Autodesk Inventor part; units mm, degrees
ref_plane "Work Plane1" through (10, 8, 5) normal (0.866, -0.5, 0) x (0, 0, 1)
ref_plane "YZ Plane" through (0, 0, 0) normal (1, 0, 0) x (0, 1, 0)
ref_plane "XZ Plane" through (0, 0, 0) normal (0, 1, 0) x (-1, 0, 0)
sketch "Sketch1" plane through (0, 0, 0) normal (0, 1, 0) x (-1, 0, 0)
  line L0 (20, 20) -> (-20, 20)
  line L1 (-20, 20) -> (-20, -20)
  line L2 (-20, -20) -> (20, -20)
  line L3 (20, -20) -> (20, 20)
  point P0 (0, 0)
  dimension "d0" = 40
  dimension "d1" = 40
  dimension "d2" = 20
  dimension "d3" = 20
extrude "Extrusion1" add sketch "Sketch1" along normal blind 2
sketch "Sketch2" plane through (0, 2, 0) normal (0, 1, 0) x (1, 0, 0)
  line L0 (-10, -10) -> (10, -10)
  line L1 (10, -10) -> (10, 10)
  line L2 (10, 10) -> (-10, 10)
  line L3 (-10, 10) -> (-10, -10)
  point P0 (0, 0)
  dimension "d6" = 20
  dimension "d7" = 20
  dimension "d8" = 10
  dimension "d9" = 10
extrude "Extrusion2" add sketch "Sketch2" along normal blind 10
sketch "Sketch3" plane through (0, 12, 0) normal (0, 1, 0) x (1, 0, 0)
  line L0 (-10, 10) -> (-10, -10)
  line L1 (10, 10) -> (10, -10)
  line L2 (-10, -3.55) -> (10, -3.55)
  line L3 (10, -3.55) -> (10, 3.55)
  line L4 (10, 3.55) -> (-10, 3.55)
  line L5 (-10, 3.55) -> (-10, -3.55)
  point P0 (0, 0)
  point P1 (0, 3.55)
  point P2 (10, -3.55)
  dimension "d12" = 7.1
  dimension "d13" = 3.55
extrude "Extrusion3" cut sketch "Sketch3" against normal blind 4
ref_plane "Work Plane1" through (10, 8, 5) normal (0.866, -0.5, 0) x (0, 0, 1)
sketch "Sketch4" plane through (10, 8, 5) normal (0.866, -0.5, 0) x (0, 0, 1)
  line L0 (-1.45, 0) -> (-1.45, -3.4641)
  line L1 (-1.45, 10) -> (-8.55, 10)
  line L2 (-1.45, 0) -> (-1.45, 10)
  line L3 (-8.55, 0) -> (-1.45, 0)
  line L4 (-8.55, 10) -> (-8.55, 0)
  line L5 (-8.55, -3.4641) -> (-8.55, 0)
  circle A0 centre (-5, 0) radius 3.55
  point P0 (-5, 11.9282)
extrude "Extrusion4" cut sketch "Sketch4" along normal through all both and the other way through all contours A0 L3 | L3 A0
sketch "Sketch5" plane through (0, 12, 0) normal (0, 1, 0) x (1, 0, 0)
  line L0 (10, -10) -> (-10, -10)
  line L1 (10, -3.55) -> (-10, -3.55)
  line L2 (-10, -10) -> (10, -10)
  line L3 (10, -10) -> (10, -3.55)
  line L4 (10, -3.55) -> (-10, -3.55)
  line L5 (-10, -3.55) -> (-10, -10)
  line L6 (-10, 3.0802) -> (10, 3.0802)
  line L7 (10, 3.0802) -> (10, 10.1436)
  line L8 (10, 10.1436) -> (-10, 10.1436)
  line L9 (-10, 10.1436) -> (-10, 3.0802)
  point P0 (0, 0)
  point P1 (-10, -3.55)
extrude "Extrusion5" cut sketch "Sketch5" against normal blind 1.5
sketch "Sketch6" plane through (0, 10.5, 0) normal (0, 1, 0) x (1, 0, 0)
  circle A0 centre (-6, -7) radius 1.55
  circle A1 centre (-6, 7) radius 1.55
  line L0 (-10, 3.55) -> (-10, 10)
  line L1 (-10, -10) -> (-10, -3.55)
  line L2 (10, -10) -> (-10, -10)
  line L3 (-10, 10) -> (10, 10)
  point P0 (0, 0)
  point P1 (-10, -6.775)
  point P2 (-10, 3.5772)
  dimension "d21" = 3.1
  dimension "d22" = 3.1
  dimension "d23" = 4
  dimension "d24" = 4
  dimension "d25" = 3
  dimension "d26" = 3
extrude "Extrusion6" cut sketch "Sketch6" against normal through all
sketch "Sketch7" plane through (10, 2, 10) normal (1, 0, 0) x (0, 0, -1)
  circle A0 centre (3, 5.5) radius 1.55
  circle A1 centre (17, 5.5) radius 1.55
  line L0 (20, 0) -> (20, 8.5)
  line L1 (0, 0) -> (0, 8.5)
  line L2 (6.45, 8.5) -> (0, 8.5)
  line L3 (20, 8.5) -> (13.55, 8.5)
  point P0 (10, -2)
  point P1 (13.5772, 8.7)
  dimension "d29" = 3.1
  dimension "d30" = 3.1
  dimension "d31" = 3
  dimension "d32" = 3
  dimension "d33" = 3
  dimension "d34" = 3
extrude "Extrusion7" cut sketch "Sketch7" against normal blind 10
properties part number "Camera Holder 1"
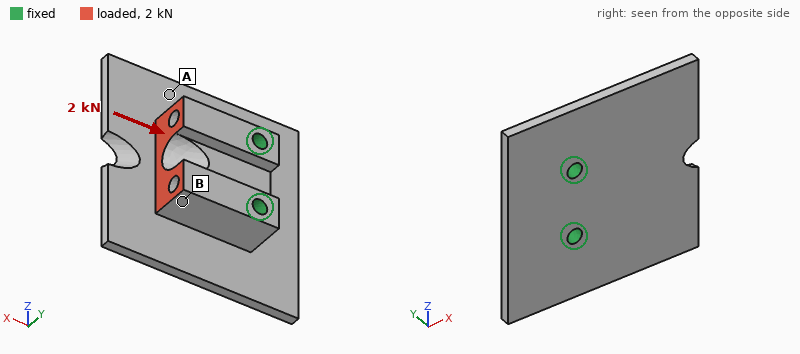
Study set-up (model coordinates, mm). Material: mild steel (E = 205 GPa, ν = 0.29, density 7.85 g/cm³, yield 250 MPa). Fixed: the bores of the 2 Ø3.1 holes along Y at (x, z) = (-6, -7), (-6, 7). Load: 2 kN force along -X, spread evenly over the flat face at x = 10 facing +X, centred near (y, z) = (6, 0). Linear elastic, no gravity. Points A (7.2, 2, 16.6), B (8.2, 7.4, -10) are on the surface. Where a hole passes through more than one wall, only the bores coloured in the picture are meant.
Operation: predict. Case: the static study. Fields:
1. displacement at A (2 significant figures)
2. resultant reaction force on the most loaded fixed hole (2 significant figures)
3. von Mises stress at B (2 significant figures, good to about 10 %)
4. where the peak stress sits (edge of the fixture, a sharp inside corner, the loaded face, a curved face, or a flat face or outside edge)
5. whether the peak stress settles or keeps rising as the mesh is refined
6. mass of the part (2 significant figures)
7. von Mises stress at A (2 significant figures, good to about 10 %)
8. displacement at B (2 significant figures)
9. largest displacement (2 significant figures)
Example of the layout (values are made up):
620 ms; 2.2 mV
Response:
0.44 µm; 1.0 kN; 18 MPa; edge of the fixture; keeps rising; 46 g; 2.5 MPa; 1.3 µm; 2.3 µm
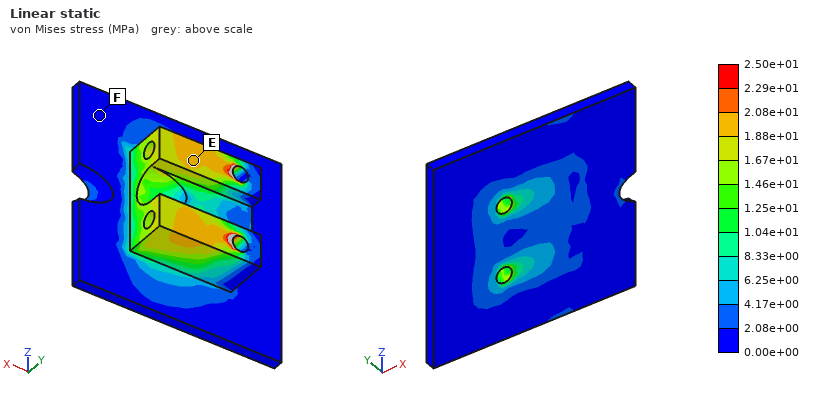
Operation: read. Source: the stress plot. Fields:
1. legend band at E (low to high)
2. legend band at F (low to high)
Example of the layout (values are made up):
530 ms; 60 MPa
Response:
1.88e+01 to 2.08e+01 MPa; 0.00e+00 to 2.08e+00 MPa
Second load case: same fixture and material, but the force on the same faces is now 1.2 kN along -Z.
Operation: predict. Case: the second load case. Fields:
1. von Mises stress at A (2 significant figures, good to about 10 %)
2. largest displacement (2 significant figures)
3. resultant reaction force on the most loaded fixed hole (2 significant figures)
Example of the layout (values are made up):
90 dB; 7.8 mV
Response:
4.4 MPa; 4.6 µm; 1.3 kN
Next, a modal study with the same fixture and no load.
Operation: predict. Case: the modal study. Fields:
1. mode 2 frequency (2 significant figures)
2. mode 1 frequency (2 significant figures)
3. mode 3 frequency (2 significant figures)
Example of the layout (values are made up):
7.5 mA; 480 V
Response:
8700 Hz; 8600 Hz; 9700 Hz
